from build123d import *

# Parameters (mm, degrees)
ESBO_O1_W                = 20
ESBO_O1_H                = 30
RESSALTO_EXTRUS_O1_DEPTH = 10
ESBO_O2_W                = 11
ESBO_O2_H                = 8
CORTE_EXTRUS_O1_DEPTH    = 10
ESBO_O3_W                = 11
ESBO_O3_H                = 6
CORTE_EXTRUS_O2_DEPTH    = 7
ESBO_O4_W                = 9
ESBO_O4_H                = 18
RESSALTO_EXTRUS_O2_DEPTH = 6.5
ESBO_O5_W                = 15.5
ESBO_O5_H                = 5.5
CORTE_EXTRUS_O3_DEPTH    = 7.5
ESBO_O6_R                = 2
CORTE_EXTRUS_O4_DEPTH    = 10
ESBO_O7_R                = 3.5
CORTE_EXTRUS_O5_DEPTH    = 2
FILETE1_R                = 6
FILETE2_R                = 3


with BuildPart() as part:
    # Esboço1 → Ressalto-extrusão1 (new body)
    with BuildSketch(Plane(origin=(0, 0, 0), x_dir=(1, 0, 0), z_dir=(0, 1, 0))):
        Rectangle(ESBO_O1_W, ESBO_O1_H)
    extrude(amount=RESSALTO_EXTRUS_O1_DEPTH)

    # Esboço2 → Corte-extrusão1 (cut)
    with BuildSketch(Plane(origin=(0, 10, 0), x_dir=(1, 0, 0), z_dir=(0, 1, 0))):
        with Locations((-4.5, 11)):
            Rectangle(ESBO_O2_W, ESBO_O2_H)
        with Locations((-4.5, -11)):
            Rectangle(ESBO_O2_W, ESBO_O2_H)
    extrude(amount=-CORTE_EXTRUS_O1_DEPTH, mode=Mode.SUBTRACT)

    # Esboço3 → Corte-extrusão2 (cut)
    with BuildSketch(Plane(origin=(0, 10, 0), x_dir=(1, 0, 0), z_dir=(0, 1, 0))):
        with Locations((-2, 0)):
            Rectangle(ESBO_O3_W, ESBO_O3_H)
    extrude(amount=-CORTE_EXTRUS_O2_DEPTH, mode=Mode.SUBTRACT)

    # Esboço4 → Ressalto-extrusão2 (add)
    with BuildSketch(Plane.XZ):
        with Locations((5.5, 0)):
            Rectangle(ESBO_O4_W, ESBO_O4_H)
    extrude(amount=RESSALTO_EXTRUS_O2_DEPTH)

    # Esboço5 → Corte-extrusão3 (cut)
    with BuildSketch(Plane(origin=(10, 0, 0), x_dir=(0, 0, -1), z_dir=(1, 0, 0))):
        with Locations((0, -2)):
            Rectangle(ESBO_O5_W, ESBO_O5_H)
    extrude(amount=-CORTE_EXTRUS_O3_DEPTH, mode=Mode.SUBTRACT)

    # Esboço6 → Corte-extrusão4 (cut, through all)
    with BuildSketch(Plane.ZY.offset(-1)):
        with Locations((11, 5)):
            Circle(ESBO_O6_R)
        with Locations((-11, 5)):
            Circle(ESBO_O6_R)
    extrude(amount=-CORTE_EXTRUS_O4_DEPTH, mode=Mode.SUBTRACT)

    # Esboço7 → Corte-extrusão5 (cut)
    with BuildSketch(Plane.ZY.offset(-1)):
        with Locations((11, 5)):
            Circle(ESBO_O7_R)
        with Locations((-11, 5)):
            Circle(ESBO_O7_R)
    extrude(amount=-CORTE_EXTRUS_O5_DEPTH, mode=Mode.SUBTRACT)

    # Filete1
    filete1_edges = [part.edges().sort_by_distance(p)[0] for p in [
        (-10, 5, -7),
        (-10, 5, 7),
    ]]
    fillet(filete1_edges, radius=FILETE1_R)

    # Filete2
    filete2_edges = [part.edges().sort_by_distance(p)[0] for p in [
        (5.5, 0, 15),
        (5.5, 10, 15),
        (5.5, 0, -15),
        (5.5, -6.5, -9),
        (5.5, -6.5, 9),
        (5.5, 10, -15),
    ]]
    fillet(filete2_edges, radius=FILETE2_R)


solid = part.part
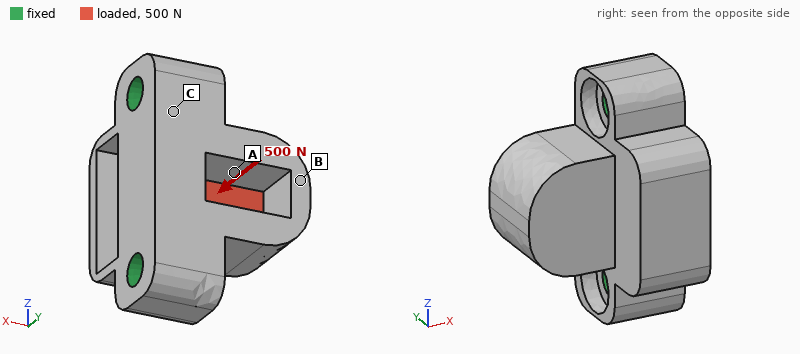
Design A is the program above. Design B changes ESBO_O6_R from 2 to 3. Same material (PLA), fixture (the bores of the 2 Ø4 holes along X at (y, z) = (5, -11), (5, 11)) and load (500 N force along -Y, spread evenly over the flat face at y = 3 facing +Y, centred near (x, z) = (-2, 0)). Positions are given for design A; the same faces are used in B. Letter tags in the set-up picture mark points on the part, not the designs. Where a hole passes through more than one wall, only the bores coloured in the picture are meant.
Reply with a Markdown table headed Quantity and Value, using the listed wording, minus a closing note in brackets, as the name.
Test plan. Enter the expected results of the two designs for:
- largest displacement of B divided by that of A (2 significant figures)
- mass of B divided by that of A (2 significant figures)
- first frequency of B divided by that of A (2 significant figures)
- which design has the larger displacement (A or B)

| Quantity | Value |
|---|---|
| largest displacement of B divided by that of A | 0.77 |
| mass of B divided by that of A | 0.94 |
| first frequency of B divided by that of A | 1.2 |
| which design has the larger displacement | A |
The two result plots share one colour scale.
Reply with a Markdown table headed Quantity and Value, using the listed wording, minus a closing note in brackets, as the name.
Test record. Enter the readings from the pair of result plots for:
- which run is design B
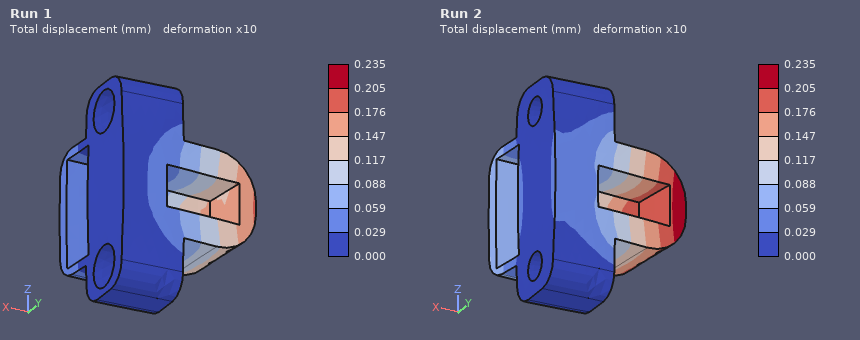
| Quantity | Value |
|---|---|
| which run is design B | Run 1 |
